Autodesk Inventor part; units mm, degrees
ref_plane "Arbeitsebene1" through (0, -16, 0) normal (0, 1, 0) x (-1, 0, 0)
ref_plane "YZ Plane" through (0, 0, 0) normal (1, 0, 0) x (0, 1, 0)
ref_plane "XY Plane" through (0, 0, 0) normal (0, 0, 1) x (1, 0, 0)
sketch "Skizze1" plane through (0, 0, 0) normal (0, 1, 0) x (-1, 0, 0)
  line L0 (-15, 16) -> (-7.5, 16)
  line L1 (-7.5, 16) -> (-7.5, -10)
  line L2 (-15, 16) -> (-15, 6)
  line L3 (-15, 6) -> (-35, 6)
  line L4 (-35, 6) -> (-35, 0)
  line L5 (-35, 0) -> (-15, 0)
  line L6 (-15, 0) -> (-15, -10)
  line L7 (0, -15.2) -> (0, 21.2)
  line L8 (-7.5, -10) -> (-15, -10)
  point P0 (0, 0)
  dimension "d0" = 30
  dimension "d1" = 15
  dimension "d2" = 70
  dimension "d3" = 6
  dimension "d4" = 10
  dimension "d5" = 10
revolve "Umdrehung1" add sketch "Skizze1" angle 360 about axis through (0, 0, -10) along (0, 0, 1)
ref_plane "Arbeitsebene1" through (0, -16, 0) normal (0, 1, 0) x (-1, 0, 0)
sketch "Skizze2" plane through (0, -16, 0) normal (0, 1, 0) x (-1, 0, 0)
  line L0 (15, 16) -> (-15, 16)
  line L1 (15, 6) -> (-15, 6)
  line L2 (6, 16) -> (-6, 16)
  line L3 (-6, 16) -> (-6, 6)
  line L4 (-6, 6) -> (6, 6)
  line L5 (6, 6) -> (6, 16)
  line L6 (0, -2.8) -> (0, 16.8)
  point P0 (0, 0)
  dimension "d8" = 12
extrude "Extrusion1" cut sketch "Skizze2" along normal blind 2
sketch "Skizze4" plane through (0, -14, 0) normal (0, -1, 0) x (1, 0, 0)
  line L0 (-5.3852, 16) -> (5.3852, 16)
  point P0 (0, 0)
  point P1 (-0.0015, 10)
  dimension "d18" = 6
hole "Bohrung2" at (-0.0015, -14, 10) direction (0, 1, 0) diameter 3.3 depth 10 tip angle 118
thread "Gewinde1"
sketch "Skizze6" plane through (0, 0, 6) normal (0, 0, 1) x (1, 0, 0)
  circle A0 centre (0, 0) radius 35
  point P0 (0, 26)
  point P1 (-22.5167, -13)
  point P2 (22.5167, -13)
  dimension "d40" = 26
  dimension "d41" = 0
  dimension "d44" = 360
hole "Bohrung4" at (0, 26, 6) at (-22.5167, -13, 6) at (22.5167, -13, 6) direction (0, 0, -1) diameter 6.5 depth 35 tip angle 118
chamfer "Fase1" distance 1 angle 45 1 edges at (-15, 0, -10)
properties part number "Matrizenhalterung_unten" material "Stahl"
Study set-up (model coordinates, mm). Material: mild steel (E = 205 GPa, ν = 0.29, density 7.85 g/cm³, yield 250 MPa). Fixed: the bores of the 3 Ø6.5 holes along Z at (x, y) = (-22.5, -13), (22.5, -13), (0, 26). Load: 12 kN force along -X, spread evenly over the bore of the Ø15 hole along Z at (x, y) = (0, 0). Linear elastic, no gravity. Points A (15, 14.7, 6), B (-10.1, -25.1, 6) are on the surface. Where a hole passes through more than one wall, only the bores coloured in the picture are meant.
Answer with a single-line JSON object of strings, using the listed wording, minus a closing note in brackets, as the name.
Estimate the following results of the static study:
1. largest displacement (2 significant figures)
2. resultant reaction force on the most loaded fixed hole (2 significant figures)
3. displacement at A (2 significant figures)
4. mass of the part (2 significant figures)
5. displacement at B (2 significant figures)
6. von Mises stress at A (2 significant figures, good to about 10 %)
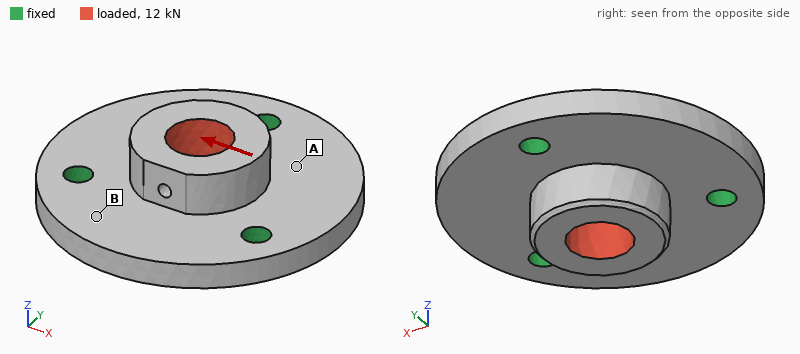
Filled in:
{"largest displacement": "5.1 µm", "resultant reaction force on the most loaded fixed hole": "4.2 kN", "displacement at A": "2.8 µm", "mass of the part": "250 g", "displacement at B": "1.1 µm", "von Mises stress at A": "16 MPa"}
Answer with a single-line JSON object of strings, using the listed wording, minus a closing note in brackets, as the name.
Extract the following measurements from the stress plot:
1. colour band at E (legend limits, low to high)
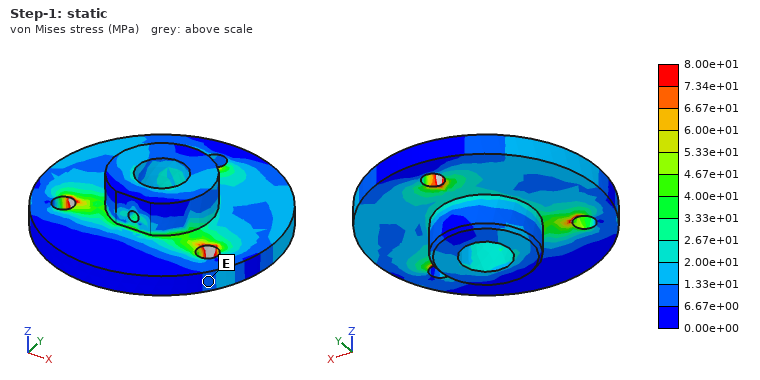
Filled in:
{"colour band at E": "6.67e+00 to 1.33e+01 MPa"}
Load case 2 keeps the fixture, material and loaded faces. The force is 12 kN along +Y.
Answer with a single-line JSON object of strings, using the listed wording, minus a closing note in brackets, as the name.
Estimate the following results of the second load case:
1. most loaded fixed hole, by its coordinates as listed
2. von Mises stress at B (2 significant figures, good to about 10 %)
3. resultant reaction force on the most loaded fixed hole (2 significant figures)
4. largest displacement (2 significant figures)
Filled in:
{"most loaded fixed hole, by its coordinates as listed": "(0, 26)", "von Mises stress at B": "16 MPa", "resultant reaction force on the most loaded fixed hole": "4.4 kN", "largest displacement": "5.4 µm"}
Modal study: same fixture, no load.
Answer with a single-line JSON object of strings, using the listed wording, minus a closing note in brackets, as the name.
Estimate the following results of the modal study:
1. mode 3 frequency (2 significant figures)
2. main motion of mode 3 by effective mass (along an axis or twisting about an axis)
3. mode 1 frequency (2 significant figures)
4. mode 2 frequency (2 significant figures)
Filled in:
{"mode 3 frequency": "11 kHz", "main motion of mode 3 by effective mass": "along Z", "mode 1 frequency": "10 kHz", "mode 2 frequency": "10 kHz"}
